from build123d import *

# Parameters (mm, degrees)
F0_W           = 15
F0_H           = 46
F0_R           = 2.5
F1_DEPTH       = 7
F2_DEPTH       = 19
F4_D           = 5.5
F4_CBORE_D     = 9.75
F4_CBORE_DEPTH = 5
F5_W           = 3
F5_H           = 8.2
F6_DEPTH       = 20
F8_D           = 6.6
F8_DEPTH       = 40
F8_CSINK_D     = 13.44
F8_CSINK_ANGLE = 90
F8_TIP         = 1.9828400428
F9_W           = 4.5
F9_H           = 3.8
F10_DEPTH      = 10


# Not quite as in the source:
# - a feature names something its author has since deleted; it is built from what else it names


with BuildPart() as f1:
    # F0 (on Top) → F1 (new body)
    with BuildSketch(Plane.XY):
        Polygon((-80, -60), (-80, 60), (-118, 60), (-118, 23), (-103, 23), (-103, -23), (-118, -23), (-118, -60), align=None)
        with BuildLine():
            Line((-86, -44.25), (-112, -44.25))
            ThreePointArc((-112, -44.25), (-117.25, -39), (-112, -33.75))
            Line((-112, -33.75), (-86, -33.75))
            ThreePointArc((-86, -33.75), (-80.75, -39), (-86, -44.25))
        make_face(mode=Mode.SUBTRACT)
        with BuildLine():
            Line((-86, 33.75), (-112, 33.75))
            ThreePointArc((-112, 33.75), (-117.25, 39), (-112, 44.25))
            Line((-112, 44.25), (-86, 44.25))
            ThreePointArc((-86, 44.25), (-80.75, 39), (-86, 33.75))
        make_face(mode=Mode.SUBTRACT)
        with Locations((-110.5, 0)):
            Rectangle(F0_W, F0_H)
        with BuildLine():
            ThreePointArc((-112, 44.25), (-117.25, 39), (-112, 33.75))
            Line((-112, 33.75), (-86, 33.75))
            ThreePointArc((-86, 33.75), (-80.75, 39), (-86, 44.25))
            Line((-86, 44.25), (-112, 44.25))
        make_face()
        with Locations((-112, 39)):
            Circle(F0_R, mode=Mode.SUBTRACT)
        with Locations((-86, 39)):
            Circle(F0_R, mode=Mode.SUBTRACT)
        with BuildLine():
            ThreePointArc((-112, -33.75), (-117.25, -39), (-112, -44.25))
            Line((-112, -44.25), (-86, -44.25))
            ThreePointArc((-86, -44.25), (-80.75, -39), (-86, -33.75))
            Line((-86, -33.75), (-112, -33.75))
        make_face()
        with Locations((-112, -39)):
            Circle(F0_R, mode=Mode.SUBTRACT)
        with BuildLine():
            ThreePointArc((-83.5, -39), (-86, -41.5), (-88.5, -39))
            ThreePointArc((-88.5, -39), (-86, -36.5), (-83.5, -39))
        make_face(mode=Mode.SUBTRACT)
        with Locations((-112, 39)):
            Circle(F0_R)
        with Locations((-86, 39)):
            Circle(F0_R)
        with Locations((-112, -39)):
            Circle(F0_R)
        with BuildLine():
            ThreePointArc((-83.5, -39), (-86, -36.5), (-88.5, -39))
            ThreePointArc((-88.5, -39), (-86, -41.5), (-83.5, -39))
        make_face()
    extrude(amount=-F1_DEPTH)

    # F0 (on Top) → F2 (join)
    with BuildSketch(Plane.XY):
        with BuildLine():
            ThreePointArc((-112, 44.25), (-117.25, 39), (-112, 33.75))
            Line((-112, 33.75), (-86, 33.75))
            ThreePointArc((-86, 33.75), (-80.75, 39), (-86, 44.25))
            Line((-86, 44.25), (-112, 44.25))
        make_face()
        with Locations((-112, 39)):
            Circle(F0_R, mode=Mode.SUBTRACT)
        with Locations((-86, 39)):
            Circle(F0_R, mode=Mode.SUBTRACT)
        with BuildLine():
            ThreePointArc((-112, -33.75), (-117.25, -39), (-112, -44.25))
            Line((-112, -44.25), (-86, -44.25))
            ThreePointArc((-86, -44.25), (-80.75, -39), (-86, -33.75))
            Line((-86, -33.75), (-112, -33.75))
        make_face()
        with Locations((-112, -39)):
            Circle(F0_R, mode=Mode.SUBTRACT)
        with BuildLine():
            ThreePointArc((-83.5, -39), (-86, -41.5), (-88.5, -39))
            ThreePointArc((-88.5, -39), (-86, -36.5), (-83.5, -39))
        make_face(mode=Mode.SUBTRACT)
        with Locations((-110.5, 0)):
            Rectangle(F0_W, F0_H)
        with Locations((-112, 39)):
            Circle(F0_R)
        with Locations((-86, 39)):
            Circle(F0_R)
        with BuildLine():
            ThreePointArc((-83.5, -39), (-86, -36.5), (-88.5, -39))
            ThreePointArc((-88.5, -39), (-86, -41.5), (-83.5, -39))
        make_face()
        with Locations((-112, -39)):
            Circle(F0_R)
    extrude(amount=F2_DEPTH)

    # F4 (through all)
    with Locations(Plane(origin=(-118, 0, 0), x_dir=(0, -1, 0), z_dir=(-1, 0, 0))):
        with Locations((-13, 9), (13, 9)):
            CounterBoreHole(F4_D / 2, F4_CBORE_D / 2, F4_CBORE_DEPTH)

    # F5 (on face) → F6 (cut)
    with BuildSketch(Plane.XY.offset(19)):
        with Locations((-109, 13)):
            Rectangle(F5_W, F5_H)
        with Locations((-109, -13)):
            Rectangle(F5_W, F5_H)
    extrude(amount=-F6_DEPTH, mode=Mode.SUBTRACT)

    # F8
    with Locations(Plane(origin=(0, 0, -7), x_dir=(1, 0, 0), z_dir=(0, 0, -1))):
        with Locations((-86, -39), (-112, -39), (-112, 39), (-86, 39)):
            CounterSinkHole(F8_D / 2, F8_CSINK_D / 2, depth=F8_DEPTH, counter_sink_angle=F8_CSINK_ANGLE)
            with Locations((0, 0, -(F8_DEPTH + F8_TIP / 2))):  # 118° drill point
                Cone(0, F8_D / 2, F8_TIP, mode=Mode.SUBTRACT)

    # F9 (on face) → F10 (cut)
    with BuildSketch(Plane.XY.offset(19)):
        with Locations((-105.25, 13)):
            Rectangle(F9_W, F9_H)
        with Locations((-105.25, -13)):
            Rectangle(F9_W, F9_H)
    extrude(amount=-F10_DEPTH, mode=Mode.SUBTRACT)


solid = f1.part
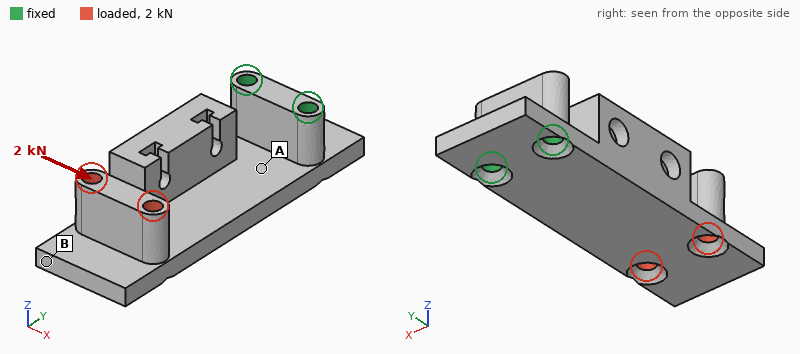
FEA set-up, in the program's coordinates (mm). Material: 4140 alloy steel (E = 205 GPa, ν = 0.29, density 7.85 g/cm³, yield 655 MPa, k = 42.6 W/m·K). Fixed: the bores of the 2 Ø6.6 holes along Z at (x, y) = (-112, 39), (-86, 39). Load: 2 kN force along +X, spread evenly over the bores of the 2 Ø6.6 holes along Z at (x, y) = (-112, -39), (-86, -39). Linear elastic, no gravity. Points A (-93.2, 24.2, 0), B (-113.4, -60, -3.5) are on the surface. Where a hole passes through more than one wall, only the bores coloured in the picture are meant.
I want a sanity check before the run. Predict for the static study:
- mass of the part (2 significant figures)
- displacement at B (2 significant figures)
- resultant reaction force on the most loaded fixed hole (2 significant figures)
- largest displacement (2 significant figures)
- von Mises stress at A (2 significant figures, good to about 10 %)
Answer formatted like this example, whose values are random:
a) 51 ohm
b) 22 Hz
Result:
a) 410 g
b) 0.10 mm
c) 5.5 kN
d) 0.15 mm
e) 74 MPa
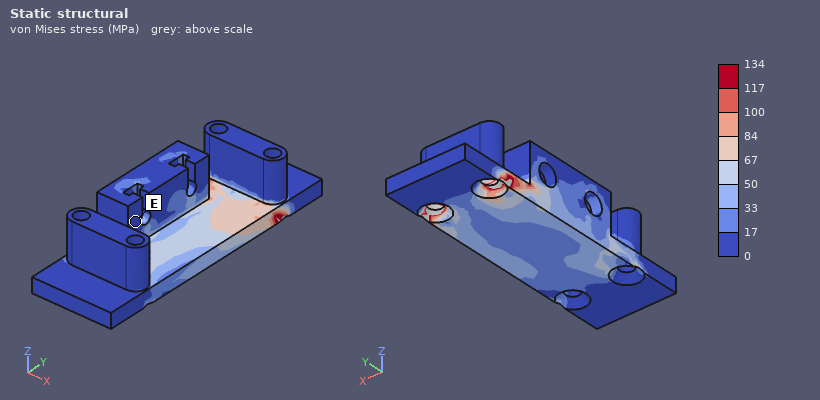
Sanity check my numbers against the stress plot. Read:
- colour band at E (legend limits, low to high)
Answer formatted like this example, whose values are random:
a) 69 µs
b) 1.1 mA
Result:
a) 0 to 17 MPa
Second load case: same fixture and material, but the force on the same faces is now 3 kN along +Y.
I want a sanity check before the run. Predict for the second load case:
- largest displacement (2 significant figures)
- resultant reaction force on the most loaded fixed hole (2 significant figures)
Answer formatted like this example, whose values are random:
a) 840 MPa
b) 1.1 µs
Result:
a) 0.43 mm
b) 1.6 kN
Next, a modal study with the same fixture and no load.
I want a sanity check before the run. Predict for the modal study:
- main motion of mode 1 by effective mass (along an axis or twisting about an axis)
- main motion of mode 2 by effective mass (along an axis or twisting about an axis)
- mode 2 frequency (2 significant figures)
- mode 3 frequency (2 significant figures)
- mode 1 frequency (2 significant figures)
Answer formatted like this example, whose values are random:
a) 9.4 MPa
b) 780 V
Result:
a) along Z
b) along X
c) 2000 Hz
d) 2900 Hz
e) 550 Hz
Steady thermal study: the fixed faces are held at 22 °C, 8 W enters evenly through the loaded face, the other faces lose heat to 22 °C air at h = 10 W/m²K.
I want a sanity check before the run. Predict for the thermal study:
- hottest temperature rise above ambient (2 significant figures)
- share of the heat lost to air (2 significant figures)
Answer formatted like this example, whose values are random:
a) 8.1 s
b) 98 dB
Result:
a) 40 K
b) 37 %
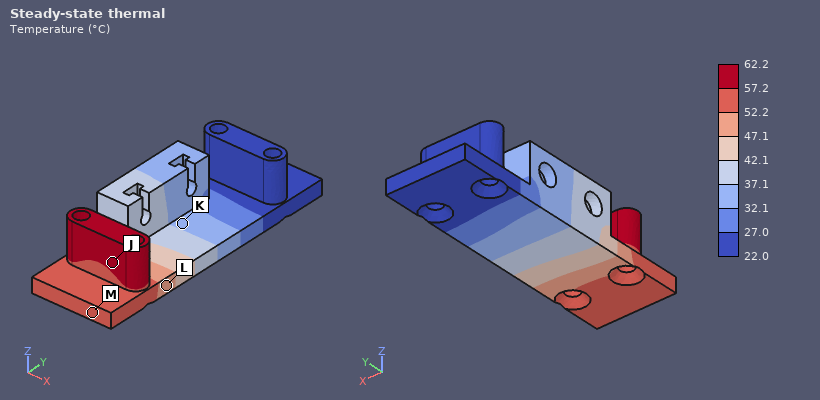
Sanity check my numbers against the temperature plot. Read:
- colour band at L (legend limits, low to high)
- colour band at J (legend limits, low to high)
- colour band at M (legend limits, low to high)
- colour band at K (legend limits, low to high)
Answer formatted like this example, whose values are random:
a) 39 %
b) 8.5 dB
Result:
a) 47.1 to 52.2 °C
b) 57.2 to 62.2 °C
c) 52.2 to 57.2 °C
d) 32.1 to 37.1 °C
